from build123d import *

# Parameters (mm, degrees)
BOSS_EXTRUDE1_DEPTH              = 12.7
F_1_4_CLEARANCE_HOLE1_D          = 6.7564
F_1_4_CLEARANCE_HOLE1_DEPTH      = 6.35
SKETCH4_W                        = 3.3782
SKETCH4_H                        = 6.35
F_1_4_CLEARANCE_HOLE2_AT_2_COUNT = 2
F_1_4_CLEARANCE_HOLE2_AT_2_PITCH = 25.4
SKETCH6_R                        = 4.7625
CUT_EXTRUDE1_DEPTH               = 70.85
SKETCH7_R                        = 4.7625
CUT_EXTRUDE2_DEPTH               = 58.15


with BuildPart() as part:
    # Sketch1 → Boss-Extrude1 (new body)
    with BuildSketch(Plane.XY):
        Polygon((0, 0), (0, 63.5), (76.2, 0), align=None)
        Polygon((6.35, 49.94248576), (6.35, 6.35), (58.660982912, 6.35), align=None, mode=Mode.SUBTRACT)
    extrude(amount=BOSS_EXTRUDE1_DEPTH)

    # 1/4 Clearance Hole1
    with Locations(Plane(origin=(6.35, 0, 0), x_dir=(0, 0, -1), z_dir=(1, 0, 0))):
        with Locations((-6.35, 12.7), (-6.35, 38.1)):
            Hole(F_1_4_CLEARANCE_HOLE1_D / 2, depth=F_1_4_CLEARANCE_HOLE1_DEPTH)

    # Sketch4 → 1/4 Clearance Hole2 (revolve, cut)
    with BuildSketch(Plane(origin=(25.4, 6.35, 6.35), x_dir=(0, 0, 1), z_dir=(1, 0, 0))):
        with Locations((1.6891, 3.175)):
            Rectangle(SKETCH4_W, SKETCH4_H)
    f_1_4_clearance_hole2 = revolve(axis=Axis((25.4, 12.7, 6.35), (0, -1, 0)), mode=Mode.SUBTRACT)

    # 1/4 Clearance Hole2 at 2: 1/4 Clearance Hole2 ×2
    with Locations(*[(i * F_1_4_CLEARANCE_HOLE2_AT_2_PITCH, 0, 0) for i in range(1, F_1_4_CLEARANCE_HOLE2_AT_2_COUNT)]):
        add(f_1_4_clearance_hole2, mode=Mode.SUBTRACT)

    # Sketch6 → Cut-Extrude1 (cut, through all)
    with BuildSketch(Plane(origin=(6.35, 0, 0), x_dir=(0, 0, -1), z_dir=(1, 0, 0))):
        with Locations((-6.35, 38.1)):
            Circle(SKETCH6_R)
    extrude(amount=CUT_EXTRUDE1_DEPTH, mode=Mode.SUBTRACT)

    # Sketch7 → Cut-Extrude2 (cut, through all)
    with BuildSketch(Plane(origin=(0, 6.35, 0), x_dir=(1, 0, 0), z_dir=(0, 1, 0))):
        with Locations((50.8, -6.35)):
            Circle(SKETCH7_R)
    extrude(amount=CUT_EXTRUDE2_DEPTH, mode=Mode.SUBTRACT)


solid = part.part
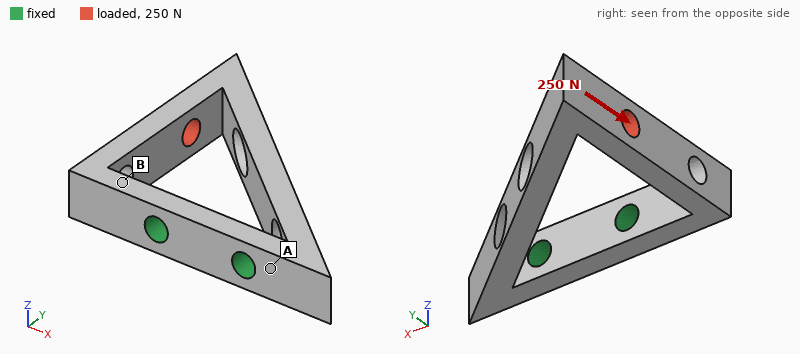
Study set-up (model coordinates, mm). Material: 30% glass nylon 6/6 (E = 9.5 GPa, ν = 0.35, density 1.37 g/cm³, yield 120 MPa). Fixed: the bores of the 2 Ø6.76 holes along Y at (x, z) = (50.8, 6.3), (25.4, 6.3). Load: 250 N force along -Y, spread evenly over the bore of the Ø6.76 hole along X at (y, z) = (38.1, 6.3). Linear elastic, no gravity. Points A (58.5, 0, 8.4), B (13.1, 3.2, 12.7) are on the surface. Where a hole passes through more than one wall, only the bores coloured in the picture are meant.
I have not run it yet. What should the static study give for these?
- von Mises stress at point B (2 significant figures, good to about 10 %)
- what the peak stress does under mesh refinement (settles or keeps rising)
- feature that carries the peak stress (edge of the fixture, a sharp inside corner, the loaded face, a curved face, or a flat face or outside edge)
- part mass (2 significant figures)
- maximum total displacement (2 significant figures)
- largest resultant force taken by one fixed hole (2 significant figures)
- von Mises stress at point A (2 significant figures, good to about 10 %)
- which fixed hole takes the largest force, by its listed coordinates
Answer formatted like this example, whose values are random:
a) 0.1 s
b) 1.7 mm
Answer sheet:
a) 11 MPa
b) keeps rising
c) edge of the fixture
d) 19 g
e) 0.31 mm
f) 270 N
g) 4.5 MPa
h) (25.4, 6.3)
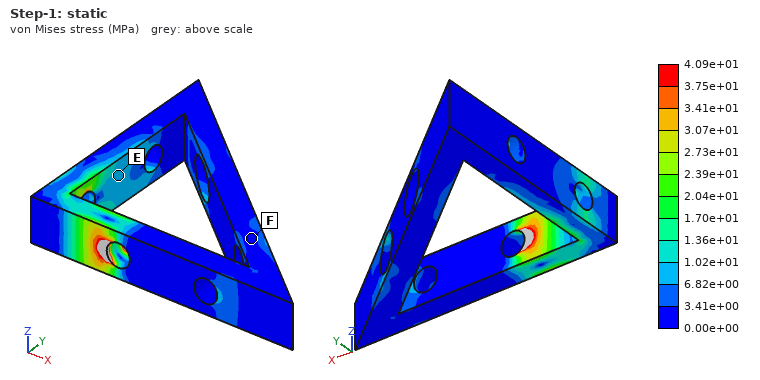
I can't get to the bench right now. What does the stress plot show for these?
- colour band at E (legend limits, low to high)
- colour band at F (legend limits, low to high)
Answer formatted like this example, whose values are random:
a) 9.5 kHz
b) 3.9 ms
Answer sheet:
a) 6.82e+00 to 1.02e+01 MPa
b) 0.00e+00 to 3.41e+00 MPa
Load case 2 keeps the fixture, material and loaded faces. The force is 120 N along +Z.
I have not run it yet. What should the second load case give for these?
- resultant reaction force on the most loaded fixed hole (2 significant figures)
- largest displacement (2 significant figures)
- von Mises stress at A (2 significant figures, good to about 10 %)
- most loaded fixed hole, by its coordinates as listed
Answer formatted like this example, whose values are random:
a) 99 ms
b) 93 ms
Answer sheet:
a) 110 N
b) 1.1 mm
c) 15 MPa
d) (25.4, 6.3)
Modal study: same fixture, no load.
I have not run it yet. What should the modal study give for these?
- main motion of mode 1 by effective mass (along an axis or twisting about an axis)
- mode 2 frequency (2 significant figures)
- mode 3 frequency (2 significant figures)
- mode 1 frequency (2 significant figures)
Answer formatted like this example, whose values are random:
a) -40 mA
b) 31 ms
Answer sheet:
a) along Z
b) 1200 Hz
c) 2700 Hz
d) 690 Hz
